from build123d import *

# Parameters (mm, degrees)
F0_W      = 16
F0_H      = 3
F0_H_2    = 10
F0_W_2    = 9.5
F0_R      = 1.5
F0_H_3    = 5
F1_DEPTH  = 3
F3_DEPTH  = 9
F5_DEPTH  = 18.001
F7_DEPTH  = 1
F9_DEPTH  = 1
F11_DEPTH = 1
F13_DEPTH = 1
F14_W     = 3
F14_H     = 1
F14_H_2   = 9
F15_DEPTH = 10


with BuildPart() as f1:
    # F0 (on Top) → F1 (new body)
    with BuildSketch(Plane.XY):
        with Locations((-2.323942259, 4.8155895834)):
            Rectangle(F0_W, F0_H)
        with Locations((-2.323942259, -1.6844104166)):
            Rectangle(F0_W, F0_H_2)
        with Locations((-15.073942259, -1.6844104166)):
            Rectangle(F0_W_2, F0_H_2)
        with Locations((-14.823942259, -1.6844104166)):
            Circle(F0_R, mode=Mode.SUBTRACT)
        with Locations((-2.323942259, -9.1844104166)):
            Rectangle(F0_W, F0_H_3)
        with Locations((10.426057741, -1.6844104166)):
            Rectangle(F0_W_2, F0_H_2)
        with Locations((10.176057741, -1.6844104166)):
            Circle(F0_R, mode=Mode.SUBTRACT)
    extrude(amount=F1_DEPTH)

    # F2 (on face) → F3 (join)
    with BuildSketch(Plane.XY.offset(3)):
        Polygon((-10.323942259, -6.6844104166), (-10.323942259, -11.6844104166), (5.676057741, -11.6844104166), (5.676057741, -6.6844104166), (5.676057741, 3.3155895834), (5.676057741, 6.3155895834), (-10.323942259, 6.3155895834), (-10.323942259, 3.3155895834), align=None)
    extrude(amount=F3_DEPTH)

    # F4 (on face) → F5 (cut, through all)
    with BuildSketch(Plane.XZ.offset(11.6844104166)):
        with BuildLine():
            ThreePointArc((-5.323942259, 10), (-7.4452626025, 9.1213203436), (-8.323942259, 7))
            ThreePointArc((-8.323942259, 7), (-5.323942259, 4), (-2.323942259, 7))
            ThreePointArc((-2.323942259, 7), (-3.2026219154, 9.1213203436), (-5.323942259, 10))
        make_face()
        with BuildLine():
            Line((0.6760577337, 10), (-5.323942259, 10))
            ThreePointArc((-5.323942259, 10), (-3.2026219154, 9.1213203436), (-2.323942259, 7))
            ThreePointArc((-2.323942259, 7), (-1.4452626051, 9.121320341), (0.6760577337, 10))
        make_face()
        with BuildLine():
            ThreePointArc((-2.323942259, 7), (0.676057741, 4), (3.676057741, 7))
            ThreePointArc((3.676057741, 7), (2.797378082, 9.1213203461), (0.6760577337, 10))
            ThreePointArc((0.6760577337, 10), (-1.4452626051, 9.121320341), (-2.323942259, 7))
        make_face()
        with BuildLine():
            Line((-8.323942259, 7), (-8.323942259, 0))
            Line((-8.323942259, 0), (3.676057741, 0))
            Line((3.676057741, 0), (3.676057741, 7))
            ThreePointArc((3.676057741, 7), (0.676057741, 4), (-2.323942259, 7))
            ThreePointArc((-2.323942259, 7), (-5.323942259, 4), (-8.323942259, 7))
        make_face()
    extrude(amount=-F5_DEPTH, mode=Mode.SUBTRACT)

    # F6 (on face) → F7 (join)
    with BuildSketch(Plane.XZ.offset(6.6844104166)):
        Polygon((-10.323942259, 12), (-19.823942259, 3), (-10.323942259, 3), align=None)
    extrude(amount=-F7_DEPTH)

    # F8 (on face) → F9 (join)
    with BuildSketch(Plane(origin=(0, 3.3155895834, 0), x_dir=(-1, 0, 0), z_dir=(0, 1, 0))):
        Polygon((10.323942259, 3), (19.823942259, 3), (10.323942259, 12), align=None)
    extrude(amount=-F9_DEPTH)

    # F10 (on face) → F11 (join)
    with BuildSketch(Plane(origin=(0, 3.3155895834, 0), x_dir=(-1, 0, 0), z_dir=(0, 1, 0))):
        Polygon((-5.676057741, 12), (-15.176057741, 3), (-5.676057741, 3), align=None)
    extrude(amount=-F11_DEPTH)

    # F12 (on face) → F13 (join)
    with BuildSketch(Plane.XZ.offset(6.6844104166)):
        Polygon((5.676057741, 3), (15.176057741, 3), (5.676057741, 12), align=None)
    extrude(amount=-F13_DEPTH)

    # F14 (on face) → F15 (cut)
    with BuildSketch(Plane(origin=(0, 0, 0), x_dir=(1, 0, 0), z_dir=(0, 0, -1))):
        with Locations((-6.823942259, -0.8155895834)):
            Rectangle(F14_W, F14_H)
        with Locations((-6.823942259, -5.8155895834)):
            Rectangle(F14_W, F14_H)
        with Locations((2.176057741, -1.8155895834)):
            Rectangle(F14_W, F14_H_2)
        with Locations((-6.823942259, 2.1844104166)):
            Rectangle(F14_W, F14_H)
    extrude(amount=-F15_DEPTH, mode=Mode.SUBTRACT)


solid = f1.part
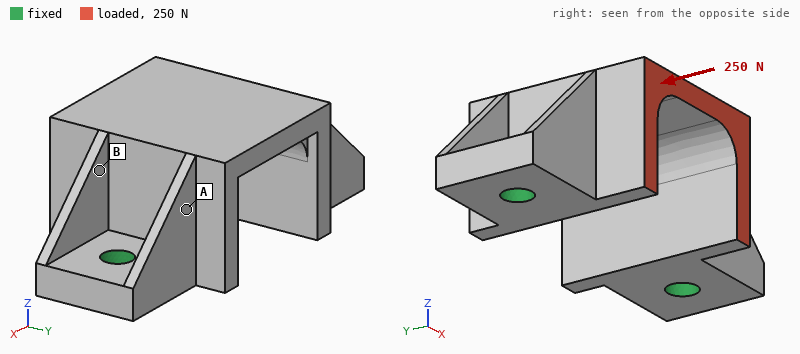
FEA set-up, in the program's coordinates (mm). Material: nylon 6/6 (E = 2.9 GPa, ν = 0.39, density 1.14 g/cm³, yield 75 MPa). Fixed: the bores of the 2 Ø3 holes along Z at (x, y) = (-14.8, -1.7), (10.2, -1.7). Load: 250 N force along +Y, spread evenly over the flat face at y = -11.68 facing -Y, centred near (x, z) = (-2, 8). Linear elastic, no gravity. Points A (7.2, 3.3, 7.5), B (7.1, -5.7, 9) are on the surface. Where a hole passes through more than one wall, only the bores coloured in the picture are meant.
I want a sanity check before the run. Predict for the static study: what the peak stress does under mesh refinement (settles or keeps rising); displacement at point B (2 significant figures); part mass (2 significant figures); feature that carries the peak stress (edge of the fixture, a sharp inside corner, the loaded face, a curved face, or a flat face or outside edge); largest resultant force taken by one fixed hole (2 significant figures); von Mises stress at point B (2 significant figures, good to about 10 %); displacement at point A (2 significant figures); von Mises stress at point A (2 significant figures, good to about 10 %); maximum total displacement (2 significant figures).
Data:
keeps rising
0.26 mm
2.3 g
edge of the fixture
130 N
17 MPa
0.22 mm
7.4 MPa
0.44 mm
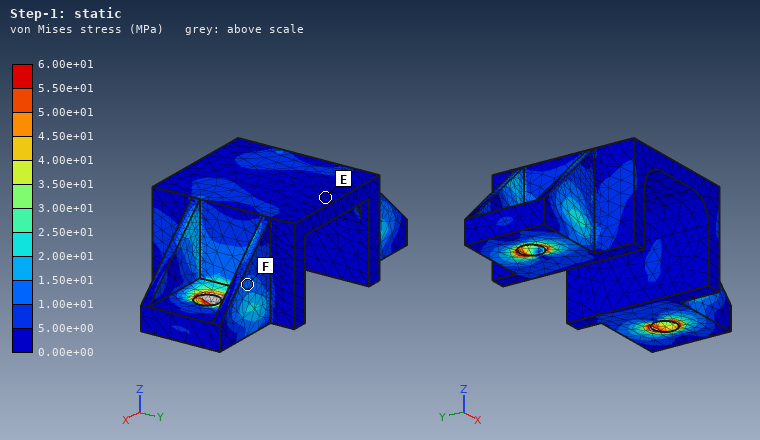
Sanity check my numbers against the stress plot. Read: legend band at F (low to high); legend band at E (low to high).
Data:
1.00e+01 to 1.50e+01 MPa
0.00e+00 to 5.00e+00 MPa
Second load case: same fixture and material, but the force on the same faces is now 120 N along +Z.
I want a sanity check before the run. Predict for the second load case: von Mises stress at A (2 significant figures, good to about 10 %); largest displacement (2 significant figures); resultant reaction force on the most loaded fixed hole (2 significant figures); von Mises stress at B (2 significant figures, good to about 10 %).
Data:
4.1 MPa
0.33 mm
67 N
12 MPa
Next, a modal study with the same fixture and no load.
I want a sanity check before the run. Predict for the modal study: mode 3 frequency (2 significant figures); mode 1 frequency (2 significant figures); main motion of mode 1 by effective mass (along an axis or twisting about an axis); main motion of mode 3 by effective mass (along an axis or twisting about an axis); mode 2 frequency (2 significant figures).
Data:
6000 Hz
3300 Hz
along Y
along X
5200 Hz
